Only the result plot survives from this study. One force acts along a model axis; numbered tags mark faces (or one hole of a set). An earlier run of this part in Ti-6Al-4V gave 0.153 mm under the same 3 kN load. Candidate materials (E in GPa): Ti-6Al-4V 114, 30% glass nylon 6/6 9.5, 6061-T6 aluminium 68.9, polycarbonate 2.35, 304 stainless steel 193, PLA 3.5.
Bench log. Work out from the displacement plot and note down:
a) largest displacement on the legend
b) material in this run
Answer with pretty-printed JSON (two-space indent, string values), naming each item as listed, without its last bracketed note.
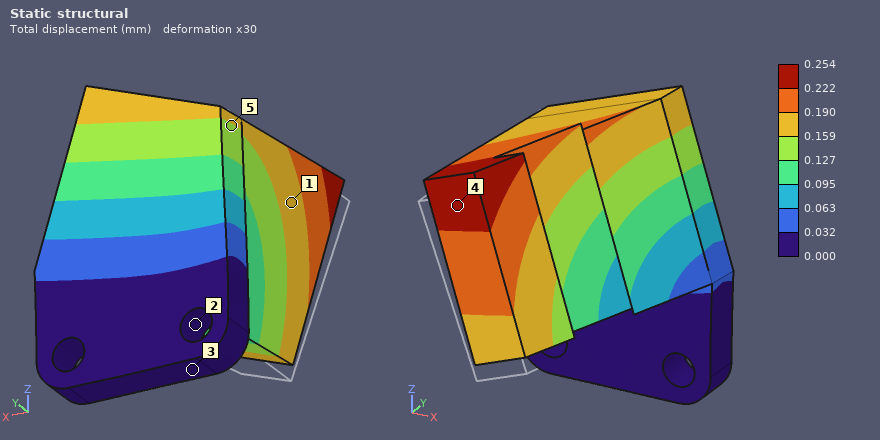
{
  "largest displacement on the legend": "0.254 mm",
  "material in this run": "6061-T6 aluminium"
}
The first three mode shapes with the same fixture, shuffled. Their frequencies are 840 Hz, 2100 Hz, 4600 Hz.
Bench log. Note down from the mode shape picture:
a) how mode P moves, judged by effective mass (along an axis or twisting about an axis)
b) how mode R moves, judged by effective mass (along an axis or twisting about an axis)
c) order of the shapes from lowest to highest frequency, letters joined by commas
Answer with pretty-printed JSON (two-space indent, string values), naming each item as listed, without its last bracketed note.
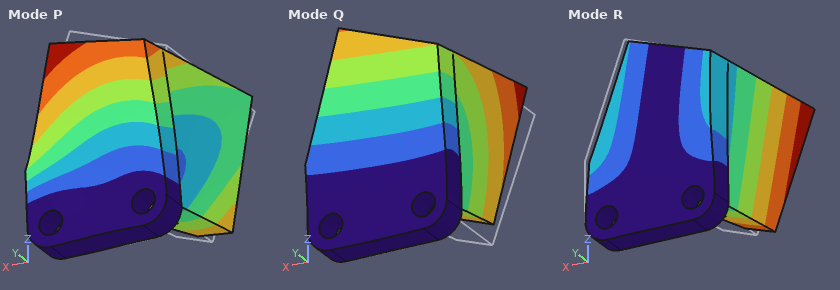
{
  "how mode P moves, judged by effective mass": "along X",
  "how mode R moves, judged by effective mass": "along X",
  "order of the shapes from lowest to highest frequency, letters joined by commas": "Q, R, P"
}
